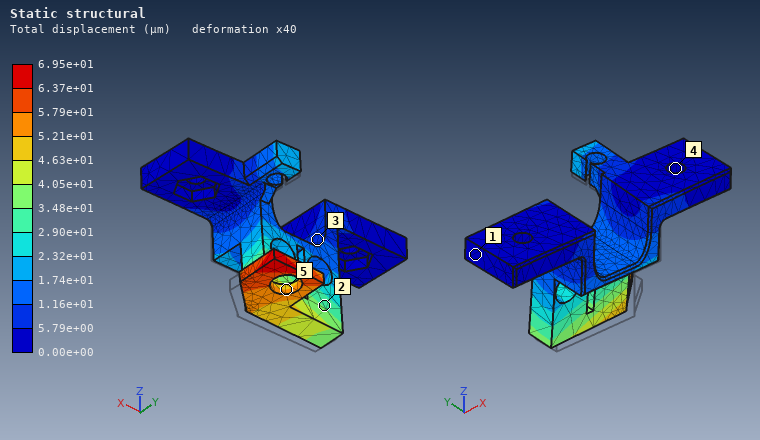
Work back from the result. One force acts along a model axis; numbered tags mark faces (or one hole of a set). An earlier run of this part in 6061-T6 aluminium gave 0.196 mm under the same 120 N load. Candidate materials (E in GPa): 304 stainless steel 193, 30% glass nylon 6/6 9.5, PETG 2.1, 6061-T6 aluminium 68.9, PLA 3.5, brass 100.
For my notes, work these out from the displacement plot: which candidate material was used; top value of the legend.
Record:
304 stainless steel
6.95e+01 µm
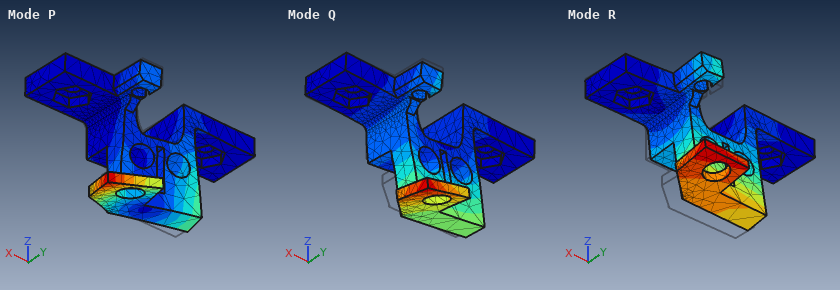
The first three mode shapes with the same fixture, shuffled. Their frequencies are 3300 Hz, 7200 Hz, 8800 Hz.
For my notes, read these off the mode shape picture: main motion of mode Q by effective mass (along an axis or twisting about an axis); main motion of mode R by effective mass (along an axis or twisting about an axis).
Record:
along X
along Y
